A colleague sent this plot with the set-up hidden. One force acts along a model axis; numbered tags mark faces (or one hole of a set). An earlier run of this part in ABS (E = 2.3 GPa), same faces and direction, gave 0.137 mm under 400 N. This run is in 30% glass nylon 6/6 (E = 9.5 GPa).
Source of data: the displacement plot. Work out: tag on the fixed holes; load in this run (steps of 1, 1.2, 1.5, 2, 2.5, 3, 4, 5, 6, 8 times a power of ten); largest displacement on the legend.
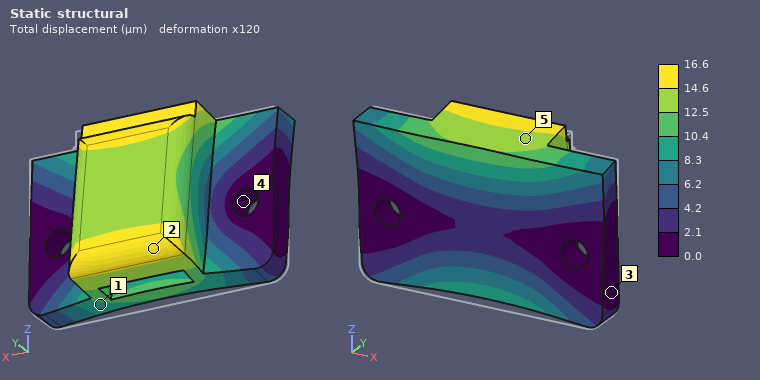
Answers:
4
200 N
16.6 µm
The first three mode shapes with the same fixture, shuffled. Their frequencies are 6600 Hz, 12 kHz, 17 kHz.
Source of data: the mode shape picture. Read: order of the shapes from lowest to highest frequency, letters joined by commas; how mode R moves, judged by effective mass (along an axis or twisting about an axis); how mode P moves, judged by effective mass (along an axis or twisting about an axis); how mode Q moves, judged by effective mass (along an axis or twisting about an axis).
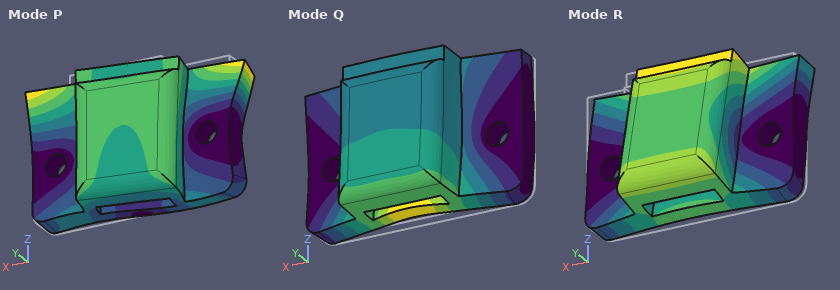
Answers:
R, Q, P
along Z
along X
along Y
